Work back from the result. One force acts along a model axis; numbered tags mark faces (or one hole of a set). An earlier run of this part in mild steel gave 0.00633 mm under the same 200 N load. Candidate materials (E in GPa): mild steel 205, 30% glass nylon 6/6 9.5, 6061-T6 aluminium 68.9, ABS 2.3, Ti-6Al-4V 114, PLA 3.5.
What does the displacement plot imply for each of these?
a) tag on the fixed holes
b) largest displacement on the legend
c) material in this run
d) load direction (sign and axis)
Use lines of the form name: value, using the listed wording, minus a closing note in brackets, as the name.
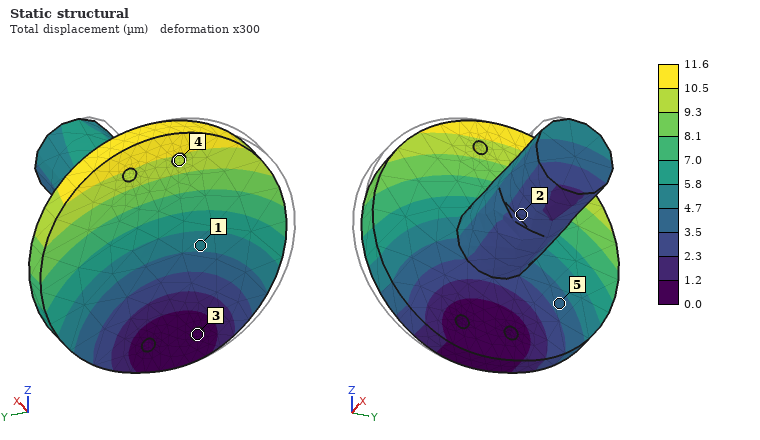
tag on the fixed holes: 3
largest displacement on the legend: 11.6 µm
material in this run: Ti-6Al-4V
load direction: +Y
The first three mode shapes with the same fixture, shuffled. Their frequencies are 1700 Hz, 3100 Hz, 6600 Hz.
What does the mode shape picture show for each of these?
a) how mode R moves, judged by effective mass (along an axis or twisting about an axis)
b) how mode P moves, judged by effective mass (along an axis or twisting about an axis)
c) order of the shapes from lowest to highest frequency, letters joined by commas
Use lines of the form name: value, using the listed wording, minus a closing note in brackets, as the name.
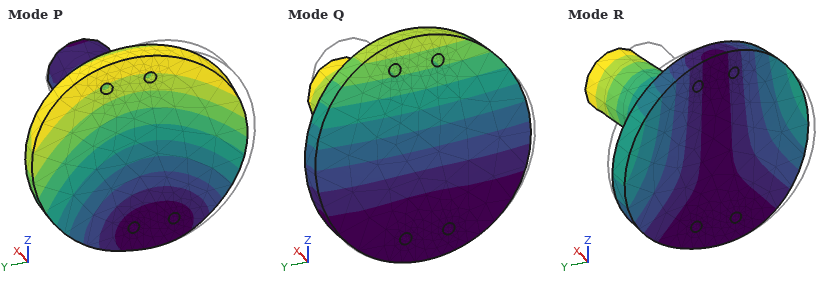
how mode R moves, judged by effective mass: along Y
how mode P moves, judged by effective mass: along Y
order of the shapes from lowest to highest frequency, letters joined by commas: Q, R, P
